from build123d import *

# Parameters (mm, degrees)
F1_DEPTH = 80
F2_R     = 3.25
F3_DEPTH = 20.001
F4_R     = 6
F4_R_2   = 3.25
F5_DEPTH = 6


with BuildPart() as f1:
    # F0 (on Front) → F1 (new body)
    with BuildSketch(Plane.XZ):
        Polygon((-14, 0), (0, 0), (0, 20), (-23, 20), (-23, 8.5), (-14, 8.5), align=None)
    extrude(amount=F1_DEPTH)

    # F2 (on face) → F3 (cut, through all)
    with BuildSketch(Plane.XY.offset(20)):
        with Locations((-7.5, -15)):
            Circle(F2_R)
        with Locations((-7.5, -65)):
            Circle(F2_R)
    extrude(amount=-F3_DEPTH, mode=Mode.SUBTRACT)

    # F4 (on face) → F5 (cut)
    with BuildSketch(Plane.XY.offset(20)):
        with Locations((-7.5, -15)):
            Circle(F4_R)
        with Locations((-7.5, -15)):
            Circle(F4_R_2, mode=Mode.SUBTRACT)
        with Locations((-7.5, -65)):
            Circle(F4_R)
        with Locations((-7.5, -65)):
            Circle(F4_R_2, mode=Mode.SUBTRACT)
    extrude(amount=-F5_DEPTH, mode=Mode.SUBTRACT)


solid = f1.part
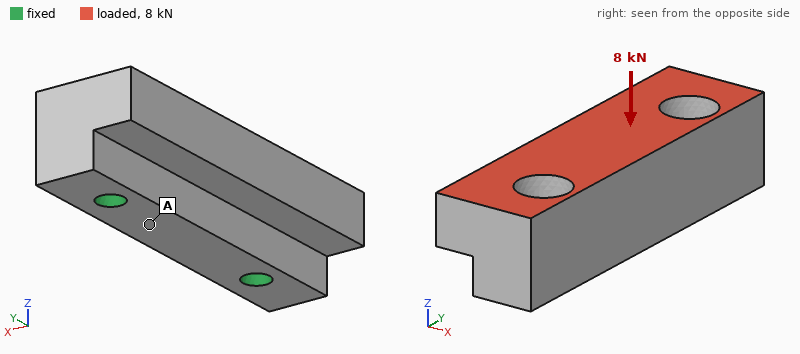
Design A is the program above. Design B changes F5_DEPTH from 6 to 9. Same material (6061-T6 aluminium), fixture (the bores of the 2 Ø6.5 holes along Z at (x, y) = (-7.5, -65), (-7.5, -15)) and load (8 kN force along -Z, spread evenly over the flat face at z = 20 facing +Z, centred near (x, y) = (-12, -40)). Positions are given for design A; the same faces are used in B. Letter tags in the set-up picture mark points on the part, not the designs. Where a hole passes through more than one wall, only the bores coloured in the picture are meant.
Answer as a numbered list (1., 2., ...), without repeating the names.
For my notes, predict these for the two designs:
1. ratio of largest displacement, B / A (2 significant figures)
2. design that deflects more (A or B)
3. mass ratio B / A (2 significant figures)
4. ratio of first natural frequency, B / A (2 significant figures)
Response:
1. 1.4
2. B
3. 0.98
4. 0.77
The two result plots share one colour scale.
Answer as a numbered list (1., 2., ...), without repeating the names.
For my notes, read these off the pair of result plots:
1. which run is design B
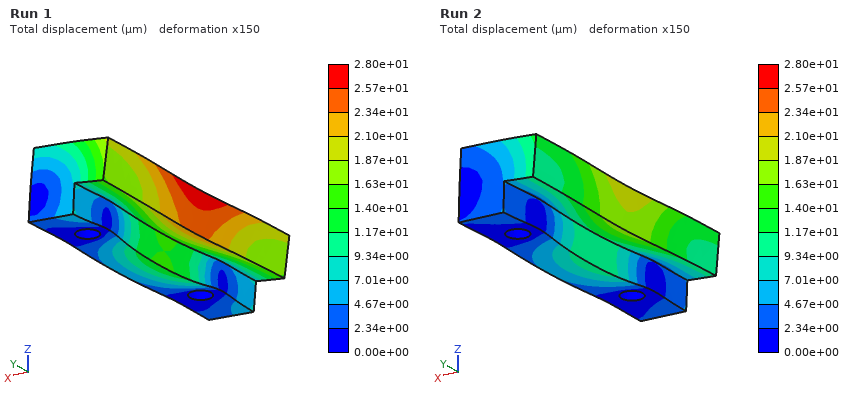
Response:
1. Run 1
